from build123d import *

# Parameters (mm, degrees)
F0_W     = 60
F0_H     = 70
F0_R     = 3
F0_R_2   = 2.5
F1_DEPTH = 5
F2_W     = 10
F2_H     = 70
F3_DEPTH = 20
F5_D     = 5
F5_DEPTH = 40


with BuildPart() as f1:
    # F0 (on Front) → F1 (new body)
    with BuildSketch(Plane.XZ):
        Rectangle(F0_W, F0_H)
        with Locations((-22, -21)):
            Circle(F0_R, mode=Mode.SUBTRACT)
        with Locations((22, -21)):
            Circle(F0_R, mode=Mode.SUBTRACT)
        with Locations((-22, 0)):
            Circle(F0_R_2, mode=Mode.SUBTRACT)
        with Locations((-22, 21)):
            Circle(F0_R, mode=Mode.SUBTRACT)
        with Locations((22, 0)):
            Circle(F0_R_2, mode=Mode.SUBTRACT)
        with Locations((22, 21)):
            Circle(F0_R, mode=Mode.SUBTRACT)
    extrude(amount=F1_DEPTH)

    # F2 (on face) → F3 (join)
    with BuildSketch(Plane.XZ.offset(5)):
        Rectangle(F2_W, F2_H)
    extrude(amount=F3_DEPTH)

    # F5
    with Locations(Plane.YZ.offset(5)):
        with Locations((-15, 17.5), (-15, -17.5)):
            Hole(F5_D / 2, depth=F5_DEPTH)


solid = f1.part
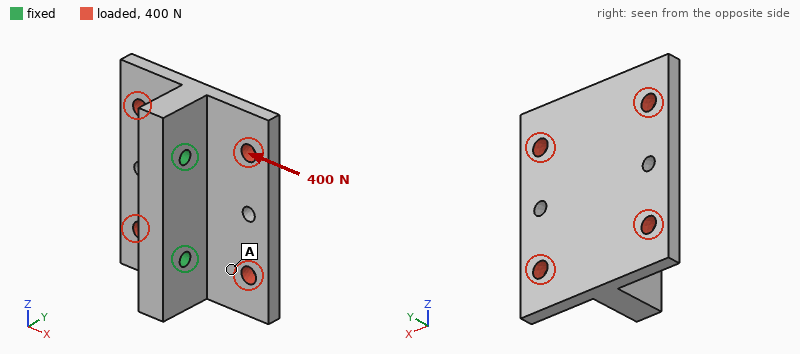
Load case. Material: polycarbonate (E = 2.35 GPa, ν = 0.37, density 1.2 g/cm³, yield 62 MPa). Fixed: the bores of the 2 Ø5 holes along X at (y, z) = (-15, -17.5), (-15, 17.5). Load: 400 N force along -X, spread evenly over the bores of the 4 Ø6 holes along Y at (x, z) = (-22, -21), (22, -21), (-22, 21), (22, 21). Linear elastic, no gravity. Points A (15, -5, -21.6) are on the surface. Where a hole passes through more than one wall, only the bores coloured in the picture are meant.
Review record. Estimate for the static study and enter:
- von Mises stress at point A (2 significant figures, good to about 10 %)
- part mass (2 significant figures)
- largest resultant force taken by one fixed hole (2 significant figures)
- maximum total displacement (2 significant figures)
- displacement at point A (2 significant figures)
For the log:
1.2 MPa
41 g
200 N
0.13 mm
0.070 mm
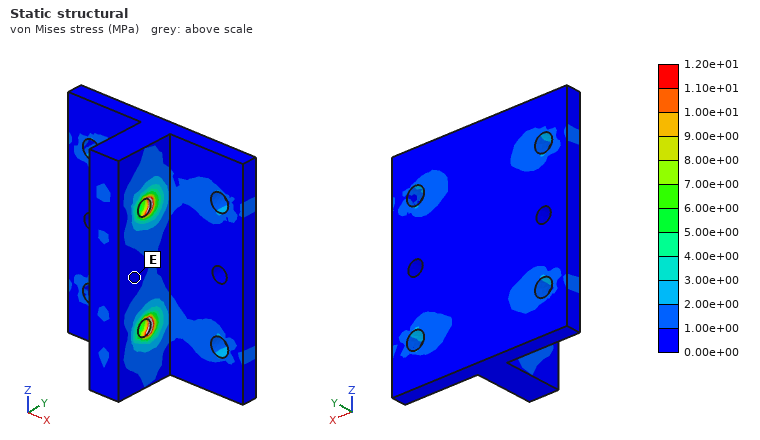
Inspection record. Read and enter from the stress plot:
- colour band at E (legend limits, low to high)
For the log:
0.00e+00 to 1.00e+00 MPa
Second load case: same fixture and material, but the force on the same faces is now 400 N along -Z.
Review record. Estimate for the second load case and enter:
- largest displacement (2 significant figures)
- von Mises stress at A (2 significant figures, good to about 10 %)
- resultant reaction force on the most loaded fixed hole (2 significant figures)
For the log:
39 µm
1.5 MPa
230 N
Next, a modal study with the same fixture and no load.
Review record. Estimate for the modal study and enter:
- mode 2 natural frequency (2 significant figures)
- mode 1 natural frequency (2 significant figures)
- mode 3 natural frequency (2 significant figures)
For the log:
1600 Hz
1200 Hz
1600 Hz
